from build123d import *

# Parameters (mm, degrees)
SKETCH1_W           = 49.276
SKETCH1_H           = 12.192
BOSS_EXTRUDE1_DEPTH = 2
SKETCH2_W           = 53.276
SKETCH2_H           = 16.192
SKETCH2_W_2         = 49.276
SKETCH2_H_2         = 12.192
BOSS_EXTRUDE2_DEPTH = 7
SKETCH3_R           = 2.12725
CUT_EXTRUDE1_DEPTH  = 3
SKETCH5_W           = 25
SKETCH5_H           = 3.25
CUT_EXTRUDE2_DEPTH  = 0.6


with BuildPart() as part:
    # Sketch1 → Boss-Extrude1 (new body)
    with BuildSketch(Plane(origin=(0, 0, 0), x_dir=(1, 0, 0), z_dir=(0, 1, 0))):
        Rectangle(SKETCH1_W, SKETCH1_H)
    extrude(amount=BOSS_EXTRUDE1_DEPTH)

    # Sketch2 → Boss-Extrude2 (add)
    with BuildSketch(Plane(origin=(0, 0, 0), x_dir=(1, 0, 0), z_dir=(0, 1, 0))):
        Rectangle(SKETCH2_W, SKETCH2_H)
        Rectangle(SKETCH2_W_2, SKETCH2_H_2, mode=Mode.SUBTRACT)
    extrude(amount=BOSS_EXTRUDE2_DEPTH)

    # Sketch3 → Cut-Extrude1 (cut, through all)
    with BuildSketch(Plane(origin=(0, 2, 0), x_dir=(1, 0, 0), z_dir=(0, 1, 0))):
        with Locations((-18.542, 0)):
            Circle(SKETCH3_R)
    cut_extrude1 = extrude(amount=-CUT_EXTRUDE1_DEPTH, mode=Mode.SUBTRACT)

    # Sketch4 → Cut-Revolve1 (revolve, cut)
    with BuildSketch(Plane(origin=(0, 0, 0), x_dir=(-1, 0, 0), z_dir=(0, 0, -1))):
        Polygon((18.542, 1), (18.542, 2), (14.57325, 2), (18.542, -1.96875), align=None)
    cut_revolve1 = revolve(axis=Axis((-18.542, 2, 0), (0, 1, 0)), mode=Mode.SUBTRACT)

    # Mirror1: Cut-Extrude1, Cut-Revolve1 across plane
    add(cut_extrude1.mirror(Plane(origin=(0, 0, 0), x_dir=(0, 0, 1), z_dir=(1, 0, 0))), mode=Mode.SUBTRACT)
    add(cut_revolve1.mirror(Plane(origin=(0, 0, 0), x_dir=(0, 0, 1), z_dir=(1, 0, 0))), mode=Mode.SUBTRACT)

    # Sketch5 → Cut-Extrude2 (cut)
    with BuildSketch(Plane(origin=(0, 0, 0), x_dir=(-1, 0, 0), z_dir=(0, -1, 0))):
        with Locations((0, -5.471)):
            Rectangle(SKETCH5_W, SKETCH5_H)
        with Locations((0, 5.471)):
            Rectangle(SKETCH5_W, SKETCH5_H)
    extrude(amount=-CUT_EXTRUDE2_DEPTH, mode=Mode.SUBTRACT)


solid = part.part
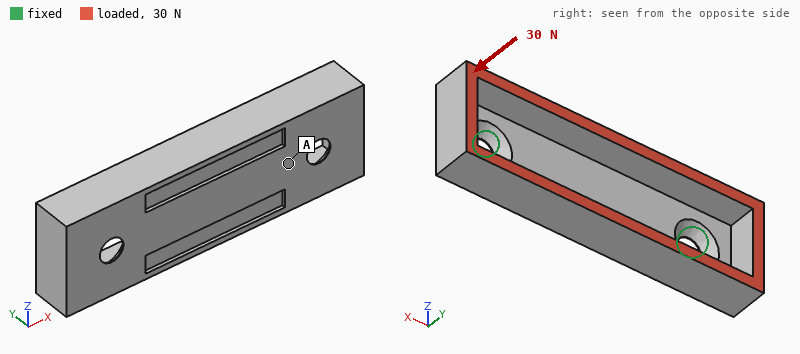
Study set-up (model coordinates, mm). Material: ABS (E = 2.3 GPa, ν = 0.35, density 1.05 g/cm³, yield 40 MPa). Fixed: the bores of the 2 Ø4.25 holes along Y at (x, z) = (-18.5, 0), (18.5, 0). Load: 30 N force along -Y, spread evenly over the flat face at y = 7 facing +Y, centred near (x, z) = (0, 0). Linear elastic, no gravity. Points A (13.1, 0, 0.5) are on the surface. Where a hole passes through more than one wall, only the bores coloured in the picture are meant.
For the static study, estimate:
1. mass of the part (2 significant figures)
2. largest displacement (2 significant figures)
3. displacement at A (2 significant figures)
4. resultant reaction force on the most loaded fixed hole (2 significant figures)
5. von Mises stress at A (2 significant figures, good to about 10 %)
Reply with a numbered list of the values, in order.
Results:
1. 3.0 g
2. 37 µm
3. 11 µm
4. 16 N
5. 1.3 MPa
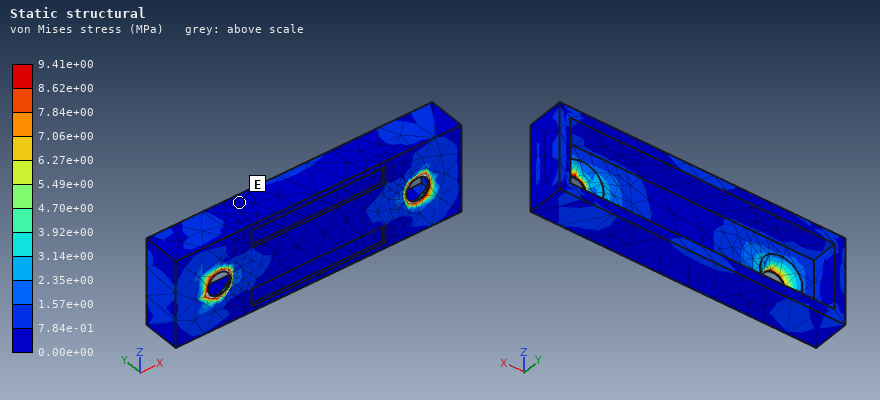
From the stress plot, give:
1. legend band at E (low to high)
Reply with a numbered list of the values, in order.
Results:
1. 0.00e+00 to 7.84e-01 MPa
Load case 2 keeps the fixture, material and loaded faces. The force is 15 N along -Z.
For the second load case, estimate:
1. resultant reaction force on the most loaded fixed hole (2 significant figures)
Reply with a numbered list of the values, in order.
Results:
1. 7.5 N
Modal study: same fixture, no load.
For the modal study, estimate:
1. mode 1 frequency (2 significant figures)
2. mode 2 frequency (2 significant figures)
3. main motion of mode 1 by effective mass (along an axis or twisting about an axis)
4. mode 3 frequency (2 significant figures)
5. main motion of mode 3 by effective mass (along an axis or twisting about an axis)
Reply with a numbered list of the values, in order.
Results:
1. 1200 Hz
2. 2000 Hz
3. along Z
4. 3000 Hz
5. along Y
